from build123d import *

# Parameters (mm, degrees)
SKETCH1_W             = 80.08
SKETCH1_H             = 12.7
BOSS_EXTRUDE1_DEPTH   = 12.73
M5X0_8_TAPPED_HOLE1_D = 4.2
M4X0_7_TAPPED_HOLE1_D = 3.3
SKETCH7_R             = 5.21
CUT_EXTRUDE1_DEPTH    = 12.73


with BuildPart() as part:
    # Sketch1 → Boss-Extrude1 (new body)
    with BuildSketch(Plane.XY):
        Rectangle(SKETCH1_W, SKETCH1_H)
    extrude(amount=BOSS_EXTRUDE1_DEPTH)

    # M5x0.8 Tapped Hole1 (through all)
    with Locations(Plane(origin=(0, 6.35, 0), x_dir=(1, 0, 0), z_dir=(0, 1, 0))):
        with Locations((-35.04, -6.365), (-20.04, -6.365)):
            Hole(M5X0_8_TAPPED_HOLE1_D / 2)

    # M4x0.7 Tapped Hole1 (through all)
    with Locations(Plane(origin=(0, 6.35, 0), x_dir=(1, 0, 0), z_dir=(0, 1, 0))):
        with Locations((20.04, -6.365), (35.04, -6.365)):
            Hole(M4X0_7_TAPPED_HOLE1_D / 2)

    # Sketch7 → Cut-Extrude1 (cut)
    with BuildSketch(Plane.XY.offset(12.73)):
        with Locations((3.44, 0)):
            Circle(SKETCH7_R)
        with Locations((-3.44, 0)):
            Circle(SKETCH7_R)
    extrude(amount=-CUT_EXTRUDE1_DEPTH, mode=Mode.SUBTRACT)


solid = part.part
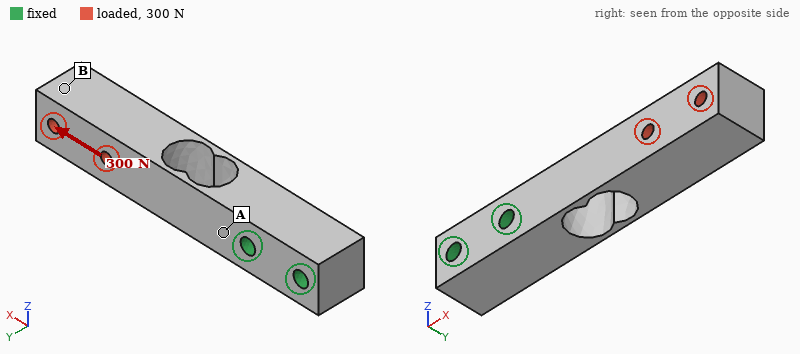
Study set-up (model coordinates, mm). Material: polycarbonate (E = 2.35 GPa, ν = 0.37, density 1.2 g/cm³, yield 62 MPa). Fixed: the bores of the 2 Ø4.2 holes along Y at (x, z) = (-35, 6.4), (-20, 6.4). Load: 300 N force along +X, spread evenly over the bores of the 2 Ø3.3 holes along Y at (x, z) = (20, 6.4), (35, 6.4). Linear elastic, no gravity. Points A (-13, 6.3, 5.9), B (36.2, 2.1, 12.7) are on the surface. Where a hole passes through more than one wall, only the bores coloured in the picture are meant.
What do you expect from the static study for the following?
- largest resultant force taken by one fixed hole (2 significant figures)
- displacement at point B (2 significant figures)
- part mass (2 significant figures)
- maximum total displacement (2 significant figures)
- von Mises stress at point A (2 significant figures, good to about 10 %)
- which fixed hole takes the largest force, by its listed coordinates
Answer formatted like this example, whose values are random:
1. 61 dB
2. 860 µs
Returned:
1. 270 N
2. 0.10 mm
3. 13 g
4. 0.11 mm
5. 4.4 MPa
6. (-20, 6.4)
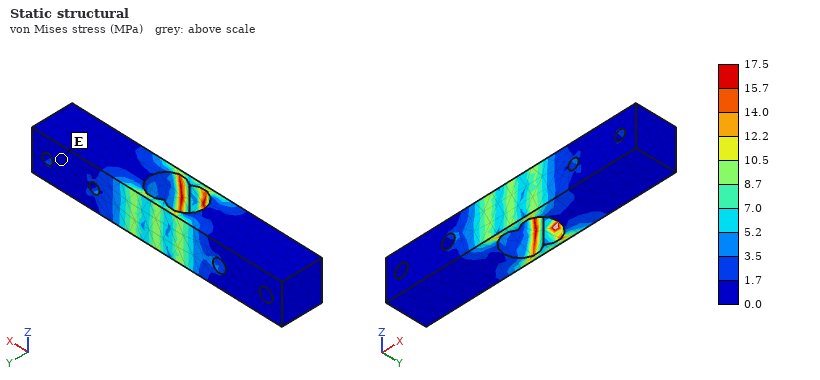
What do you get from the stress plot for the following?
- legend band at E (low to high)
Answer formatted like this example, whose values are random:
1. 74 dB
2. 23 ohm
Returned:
1. 0.0 to 1.7 MPa
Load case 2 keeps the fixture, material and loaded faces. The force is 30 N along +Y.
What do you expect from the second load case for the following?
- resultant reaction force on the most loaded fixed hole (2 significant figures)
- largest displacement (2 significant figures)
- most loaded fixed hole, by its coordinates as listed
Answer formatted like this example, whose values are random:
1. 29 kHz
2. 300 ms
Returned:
1. 42 N
2. 0.90 mm
3. (-20, 6.4)
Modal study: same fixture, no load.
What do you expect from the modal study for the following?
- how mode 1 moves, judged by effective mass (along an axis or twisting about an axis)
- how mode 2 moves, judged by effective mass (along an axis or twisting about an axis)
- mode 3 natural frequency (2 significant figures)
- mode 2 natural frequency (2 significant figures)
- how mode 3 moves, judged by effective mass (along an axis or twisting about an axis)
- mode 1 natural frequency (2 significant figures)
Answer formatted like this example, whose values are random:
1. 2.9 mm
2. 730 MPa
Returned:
1. along Y
2. along Z
3. 1800 Hz
4. 480 Hz
5. twisting about X
6. 410 Hz
